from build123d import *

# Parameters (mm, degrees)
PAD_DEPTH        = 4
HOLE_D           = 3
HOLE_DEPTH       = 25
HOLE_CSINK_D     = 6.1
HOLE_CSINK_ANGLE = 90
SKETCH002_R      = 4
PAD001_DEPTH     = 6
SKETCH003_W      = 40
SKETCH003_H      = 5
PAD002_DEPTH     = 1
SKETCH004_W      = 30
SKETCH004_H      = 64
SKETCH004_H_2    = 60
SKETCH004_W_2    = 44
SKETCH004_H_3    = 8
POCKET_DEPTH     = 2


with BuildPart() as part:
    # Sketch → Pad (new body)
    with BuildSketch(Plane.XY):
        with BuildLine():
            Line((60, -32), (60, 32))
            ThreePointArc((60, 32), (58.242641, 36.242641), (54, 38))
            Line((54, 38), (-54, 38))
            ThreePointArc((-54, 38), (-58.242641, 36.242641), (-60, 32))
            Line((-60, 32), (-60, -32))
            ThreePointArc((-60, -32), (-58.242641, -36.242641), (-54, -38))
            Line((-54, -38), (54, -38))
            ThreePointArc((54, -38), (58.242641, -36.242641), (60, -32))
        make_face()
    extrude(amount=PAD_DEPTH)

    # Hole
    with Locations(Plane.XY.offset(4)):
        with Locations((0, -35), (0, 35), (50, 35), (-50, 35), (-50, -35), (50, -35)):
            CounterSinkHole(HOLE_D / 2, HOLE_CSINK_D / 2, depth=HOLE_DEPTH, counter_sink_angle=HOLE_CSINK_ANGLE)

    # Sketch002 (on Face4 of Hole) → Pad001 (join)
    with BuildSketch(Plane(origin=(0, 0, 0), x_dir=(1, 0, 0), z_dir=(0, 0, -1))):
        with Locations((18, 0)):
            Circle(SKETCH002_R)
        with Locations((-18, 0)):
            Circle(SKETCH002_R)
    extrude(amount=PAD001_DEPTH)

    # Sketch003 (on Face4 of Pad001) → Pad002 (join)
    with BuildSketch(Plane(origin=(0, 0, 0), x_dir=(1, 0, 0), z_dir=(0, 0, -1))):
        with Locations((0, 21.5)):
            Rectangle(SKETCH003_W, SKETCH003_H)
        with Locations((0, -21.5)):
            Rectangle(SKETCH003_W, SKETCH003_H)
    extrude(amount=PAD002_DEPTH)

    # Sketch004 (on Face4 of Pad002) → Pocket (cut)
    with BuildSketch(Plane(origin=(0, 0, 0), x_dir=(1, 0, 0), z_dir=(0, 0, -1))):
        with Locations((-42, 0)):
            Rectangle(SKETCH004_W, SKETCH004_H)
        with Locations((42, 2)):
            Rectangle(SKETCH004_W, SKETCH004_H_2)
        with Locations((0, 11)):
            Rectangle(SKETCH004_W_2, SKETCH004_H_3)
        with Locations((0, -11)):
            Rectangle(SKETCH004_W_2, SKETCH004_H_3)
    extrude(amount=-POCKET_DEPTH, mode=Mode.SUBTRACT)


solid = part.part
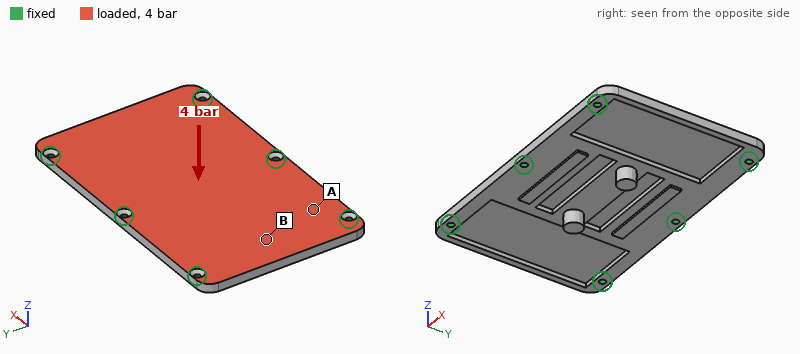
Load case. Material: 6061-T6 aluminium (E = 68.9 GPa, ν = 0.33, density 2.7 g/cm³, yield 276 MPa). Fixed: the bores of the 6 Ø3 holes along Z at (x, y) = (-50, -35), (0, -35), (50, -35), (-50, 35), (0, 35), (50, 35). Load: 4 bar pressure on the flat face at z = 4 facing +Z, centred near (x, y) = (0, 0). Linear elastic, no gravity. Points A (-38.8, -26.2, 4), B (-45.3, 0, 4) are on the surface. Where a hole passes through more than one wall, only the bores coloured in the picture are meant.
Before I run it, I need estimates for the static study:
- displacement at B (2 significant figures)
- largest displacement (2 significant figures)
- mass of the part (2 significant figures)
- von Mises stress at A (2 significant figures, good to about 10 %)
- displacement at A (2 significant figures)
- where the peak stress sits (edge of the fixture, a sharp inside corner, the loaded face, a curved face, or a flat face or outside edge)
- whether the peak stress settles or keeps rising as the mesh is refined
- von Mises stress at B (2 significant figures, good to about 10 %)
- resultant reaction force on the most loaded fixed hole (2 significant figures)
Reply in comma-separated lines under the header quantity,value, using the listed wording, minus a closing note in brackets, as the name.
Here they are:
quantity,value
displacement at B,0.31 mm
largest displacement,0.31 mm
mass of the part,76 g
von Mises stress at A,27 MPa
displacement at A,0.10 mm
where the peak stress sits,edge of the fixture
whether the peak stress settles or keeps rising as the mesh is refined,keeps rising
von Mises stress at B,71 MPa
resultant reaction force on the most loaded fixed hole,1.8 kN
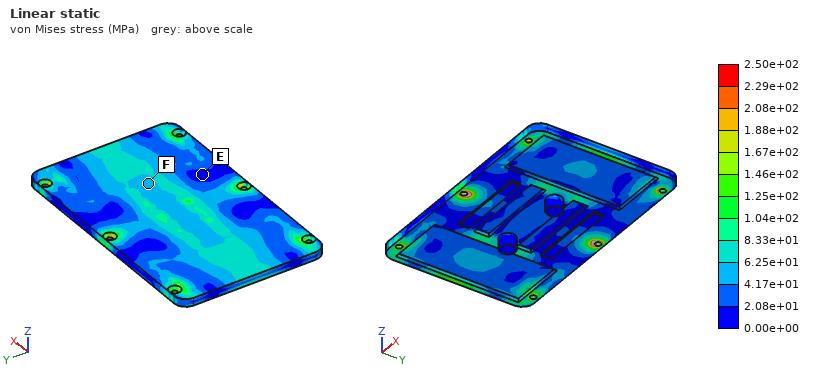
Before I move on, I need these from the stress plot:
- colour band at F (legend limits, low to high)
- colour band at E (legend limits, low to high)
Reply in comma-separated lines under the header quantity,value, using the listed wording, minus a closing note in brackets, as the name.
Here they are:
quantity,value
colour band at F,4.17e+01 to 6.25e+01 MPa
colour band at E,0.00e+00 to 2.08e+01 MPa
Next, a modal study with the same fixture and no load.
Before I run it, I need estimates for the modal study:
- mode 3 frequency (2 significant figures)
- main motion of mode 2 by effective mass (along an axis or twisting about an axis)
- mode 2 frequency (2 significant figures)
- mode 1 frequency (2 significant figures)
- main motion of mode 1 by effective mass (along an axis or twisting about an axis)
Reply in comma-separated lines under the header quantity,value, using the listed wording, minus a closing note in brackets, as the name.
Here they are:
quantity,value
mode 3 frequency,3700 Hz
main motion of mode 2 by effective mass,twisting about Y
mode 2 frequency,2900 Hz
mode 1 frequency,2500 Hz
main motion of mode 1 by effective mass,along Z
